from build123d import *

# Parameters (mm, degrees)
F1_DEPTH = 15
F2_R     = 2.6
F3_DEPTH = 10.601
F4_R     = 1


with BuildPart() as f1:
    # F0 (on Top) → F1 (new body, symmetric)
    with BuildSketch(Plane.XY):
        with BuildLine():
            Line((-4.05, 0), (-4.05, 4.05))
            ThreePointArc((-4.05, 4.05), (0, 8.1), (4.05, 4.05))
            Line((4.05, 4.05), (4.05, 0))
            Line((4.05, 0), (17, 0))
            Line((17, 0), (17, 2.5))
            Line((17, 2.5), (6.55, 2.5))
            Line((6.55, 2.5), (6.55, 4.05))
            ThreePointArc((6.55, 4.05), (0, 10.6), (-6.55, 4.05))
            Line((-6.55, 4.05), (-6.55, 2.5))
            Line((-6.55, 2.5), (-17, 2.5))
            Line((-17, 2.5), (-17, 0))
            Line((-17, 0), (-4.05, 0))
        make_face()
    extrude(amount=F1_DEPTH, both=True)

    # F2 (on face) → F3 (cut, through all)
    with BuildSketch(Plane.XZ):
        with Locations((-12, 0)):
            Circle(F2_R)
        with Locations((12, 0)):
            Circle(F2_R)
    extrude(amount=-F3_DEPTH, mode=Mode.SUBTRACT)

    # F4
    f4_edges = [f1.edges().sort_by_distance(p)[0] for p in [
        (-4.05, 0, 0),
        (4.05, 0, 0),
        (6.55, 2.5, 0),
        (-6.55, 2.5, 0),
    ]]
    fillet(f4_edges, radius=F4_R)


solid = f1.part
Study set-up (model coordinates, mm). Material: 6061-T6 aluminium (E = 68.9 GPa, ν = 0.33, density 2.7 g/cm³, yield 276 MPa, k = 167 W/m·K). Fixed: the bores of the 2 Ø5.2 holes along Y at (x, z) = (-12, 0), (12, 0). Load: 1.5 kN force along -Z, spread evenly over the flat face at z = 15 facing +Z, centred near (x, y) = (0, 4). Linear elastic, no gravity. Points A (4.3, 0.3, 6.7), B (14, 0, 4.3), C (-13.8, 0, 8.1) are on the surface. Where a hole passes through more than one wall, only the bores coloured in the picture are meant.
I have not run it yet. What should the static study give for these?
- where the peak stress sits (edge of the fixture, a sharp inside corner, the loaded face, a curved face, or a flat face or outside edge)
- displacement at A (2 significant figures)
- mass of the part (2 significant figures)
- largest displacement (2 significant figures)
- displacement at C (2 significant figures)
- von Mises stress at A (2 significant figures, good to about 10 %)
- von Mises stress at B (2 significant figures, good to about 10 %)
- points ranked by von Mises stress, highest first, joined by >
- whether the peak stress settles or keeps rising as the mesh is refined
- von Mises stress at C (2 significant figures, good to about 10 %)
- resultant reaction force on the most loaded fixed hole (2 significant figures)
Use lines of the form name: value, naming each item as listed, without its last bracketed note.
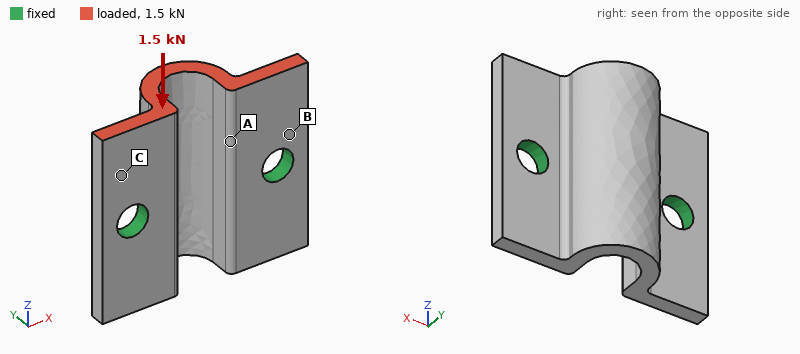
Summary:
where the peak stress sits: edge of the fixture
displacement at A: 16 µm
mass of the part: 9.0 g
largest displacement: 46 µm
displacement at C: 8.0 µm
von Mises stress at A: 9.5 MPa
von Mises stress at B: 37 MPa
points ranked by von Mises stress, highest first, joined by >: B > C > A
whether the peak stress settles or keeps rising as the mesh is refined: keeps rising
von Mises stress at C: 21 MPa
resultant reaction force on the most loaded fixed hole: 750 N
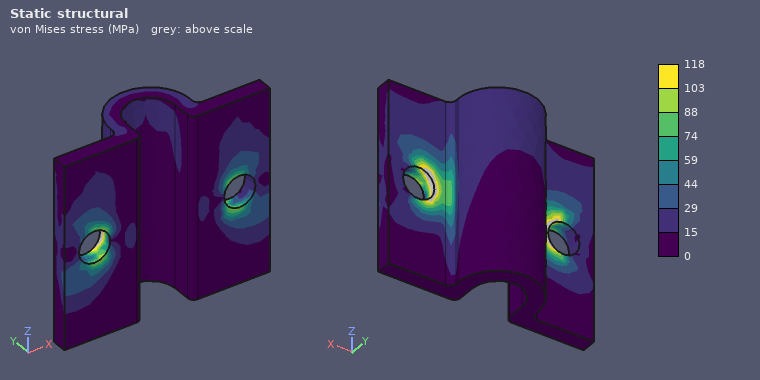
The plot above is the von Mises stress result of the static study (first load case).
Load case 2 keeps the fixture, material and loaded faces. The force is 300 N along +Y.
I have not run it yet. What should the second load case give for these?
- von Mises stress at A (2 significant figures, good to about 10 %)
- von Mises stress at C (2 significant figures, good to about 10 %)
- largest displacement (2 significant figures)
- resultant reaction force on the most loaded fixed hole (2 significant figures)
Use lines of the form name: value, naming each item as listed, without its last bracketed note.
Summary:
von Mises stress at A: 18 MPa
von Mises stress at C: 24 MPa
largest displacement: 46 µm
resultant reaction force on the most loaded fixed hole: 150 N
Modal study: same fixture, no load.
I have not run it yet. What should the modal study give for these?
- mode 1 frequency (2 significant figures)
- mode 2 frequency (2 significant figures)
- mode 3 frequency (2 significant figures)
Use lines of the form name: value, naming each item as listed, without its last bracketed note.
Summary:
mode 1 frequency: 8100 Hz
mode 2 frequency: 18 kHz
mode 3 frequency: 18 kHz
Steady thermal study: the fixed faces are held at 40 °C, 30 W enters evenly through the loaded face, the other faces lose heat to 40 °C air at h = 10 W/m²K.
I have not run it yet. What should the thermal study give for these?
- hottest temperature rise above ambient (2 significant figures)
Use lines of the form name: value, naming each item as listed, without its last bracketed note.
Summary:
hottest temperature rise above ambient: 29 K
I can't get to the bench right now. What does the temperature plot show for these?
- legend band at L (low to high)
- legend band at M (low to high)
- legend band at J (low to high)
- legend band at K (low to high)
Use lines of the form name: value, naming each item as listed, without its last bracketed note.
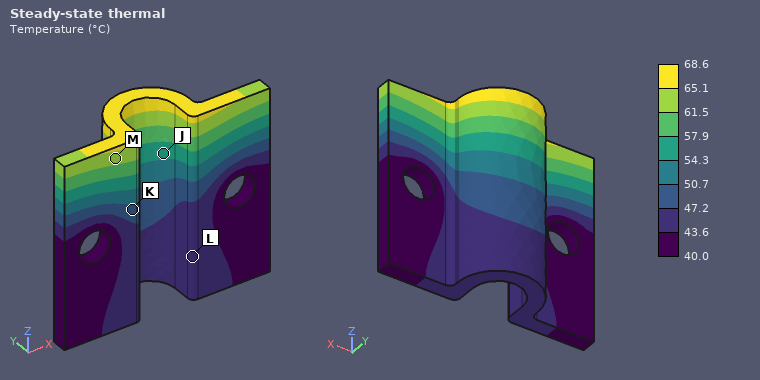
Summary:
legend band at L: 43.6 to 47.2 °C
legend band at M: 61.5 to 65.1 °C
legend band at J: 54.3 to 57.9 °C
legend band at K: 47.2 to 50.7 °C
